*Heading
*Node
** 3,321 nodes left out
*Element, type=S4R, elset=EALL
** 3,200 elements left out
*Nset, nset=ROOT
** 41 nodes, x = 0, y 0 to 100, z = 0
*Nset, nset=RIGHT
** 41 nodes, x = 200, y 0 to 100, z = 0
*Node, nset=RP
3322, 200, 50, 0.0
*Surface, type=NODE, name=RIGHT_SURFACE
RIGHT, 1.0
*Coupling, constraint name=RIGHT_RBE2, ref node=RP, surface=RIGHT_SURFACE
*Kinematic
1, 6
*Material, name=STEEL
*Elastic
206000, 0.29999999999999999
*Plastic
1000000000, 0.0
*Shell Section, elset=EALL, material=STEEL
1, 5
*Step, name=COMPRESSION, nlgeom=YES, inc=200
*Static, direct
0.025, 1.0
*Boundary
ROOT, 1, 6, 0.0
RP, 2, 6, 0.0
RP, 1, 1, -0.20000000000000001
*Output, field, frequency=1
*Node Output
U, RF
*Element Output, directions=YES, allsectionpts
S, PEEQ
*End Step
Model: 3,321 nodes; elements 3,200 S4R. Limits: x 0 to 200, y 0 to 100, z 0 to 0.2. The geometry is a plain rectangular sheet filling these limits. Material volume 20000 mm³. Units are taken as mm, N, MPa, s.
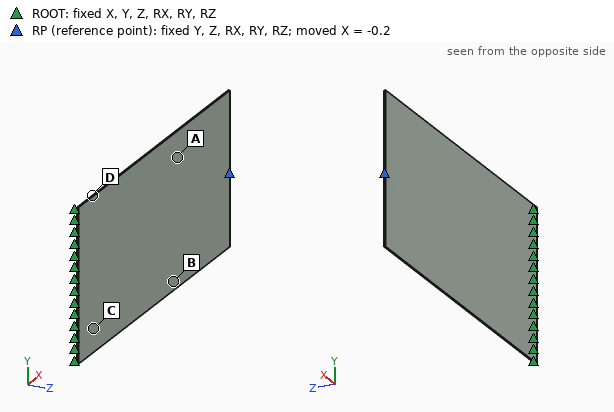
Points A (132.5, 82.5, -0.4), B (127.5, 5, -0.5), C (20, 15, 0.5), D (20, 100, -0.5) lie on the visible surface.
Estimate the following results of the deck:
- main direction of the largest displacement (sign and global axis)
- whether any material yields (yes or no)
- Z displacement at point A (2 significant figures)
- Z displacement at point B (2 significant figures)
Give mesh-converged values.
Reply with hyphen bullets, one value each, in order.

- +Z
- no
- 3.6 mm
- 3.8 mm
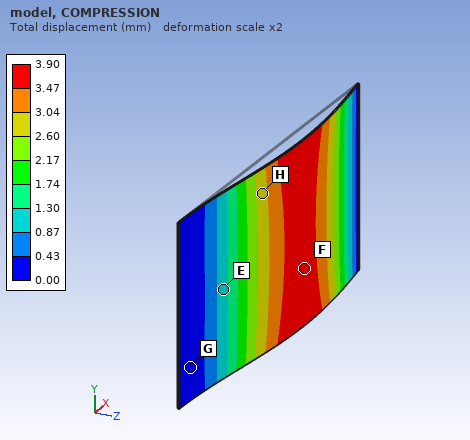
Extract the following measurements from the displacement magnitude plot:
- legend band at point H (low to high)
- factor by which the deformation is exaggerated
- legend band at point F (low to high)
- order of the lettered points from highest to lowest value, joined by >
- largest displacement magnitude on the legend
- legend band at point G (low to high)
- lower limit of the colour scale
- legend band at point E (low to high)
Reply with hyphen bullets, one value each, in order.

- 2.60 to 3.04 mm
- 2
- 3.47 to 3.90 mm
- F > H > E > G
- 3.90 mm
- 0.00 to 0.43 mm
- 0.00 mm
- 0.87 to 1.30 mm
